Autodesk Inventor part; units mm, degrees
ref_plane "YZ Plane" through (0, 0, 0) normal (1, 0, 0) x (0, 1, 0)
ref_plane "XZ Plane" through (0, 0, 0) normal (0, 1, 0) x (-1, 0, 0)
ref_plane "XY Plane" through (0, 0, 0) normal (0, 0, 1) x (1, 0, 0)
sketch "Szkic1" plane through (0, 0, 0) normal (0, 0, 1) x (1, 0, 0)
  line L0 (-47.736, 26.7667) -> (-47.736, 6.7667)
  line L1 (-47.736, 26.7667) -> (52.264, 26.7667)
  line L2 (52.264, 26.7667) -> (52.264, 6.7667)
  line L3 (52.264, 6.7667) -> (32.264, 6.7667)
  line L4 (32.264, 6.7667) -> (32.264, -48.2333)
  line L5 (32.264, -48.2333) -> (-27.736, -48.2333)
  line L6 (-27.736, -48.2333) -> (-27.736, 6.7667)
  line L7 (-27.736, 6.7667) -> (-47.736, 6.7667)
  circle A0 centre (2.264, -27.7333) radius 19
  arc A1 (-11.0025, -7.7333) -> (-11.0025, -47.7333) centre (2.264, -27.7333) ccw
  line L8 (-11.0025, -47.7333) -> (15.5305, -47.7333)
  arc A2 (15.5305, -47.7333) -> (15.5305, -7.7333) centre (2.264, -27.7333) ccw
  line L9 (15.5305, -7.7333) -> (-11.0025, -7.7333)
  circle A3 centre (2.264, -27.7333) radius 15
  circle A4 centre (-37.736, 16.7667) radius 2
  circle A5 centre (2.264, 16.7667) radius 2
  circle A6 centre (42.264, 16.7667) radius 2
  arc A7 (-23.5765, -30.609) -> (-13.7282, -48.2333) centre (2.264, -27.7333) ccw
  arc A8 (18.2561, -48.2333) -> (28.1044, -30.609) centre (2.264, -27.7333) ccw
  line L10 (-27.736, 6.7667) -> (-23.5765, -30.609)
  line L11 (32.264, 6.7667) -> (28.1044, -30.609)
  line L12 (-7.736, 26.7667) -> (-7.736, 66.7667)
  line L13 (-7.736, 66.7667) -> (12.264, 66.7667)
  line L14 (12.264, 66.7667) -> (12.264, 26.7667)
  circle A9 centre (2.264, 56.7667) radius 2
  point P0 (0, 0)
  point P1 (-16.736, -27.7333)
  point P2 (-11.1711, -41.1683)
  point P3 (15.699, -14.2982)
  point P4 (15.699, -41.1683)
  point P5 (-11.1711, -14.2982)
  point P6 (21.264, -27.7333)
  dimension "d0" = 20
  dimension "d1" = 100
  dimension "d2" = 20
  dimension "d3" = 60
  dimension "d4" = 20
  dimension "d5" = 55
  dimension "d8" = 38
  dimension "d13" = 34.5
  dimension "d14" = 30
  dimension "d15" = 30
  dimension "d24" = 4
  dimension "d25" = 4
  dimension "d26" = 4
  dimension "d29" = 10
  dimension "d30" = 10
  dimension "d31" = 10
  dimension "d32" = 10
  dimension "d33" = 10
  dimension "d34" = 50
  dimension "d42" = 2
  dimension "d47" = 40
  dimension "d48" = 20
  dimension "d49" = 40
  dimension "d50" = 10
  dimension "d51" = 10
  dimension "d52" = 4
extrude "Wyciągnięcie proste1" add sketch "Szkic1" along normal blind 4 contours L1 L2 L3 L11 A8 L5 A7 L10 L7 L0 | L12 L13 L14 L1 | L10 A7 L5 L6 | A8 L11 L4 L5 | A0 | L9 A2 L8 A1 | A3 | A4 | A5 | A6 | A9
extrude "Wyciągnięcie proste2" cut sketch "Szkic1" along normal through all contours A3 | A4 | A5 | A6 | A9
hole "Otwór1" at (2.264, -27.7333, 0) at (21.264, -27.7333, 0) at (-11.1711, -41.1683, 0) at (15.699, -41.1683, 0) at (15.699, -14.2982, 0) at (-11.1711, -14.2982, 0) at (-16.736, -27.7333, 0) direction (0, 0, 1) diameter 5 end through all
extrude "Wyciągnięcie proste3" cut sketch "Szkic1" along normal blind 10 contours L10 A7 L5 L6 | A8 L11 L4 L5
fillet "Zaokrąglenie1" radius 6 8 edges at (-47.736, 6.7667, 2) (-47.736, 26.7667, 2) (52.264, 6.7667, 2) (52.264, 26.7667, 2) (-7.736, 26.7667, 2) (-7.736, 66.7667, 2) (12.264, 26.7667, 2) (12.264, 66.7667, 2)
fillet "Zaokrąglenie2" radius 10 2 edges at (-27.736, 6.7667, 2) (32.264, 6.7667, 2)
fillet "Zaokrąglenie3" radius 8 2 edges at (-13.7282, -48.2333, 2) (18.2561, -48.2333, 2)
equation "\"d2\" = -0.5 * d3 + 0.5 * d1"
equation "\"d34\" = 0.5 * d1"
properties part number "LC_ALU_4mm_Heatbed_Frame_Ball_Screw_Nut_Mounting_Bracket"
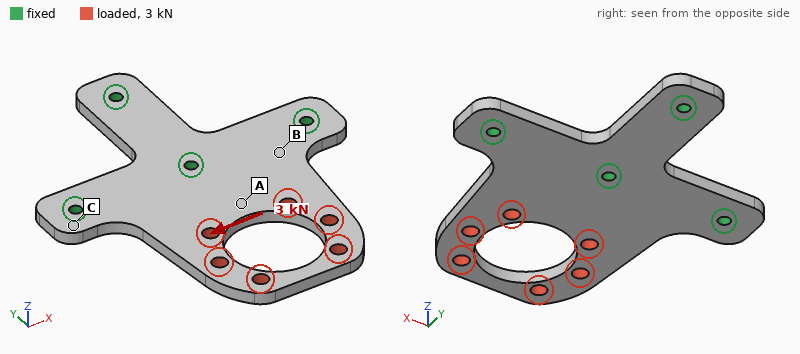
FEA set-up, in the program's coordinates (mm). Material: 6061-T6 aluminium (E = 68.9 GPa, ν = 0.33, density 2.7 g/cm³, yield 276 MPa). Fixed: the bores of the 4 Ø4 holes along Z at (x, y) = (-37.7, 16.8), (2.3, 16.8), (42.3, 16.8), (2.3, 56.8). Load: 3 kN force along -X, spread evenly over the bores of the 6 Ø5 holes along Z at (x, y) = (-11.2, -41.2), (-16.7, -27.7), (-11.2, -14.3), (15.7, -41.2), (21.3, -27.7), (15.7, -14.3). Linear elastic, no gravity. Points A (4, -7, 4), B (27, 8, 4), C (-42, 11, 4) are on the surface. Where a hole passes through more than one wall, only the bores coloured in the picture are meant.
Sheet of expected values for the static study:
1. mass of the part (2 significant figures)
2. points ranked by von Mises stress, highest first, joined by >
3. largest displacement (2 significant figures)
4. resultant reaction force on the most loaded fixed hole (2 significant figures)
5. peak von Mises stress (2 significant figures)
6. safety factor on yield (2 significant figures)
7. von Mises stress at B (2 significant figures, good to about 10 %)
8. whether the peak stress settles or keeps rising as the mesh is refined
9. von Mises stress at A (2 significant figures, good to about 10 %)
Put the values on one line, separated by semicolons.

52 g; A > B > C; 0.15 mm; 1.9 kN; 240 MPa; 1.2; 23 MPa; settles; 45 MPa
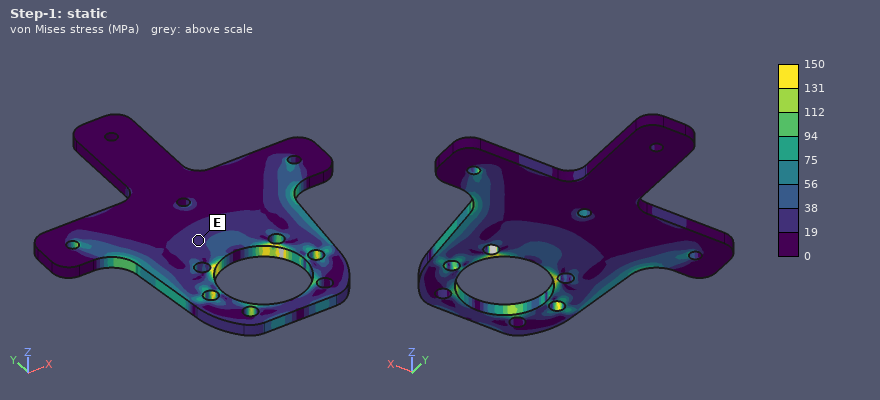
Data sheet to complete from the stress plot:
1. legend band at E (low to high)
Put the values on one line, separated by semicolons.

19 to 38 MPa
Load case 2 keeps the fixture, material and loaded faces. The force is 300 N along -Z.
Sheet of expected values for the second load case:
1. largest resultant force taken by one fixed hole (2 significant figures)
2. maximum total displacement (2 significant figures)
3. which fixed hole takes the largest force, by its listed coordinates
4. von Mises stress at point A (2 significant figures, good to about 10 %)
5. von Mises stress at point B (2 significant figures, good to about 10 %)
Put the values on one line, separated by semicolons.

320 N; 0.88 mm; (2.3, 16.8); 23 MPa; 52 MPa
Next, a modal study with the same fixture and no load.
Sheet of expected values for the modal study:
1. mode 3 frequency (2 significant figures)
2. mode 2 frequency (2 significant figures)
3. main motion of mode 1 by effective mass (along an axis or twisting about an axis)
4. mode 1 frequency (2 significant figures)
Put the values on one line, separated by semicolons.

4000 Hz; 2400 Hz; along Z; 1000 Hz
